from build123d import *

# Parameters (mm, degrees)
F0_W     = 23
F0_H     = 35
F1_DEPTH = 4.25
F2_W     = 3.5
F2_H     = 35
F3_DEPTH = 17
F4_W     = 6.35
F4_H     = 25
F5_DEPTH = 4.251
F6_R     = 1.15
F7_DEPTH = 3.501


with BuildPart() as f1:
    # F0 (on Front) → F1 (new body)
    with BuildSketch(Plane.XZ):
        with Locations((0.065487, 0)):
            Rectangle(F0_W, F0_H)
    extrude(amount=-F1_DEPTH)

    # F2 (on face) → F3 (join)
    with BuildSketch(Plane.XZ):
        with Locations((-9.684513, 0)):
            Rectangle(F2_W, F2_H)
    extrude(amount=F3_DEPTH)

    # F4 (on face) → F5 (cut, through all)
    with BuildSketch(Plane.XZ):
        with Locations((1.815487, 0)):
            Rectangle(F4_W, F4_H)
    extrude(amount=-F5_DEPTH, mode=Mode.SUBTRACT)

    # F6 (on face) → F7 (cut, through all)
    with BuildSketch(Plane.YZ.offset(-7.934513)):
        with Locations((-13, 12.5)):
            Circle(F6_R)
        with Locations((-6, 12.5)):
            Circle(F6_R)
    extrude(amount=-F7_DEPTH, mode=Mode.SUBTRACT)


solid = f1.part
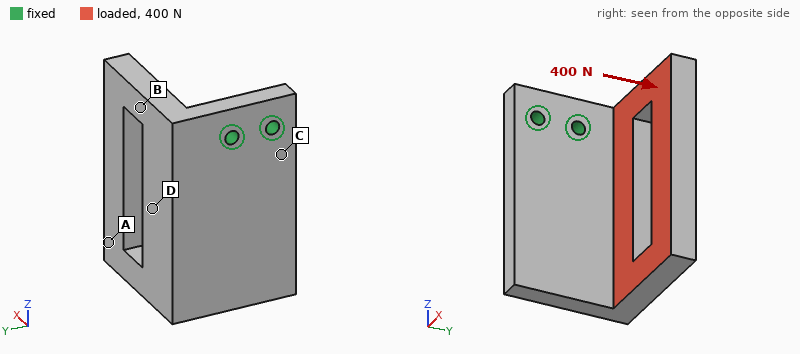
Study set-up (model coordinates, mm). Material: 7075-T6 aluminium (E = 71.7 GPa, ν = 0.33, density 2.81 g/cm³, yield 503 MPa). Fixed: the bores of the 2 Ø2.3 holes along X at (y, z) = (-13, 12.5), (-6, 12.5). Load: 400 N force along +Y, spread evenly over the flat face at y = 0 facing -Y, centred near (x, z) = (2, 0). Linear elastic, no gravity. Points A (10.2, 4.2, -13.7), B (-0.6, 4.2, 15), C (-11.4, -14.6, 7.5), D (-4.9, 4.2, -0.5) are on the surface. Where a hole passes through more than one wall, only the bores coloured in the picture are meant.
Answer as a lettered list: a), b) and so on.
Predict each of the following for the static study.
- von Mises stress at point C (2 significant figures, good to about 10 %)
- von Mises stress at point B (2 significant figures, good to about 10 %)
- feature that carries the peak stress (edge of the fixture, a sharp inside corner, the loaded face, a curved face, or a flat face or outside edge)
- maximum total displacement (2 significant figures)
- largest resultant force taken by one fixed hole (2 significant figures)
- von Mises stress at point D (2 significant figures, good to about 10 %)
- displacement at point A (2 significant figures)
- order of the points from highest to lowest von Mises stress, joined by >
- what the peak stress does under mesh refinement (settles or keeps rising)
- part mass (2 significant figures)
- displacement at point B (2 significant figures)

a) 45 MPa
b) 63 MPa
c) edge of the fixture
d) 0.27 mm
e) 680 N
f) 21 MPa
g) 0.25 mm
h) B > C > D > A
i) keeps rising
j) 13 g
k) 0.085 mm
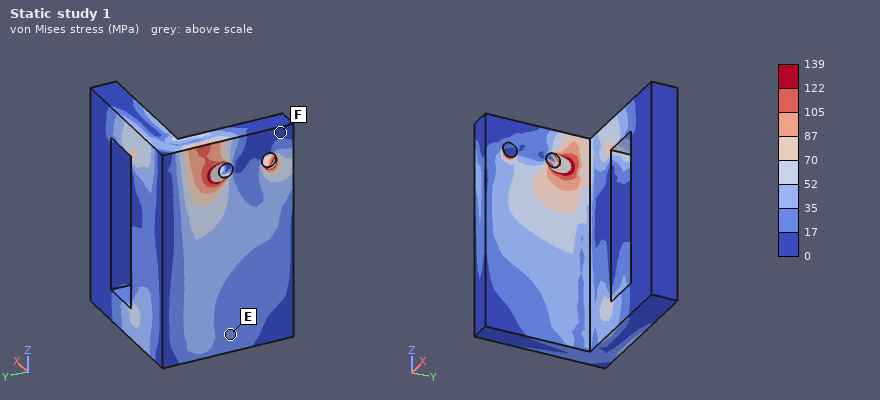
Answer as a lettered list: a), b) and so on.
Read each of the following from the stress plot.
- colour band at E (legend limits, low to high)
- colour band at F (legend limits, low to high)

a) 17 to 35 MPa
b) 0 to 17 MPa
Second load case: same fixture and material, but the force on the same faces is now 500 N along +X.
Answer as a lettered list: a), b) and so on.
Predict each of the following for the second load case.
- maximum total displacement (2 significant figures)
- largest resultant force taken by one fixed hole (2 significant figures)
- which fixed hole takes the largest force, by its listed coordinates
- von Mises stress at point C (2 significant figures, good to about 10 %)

a) 0.29 mm
b) 630 N
c) (-6, 12.5)
d) 80 MPa
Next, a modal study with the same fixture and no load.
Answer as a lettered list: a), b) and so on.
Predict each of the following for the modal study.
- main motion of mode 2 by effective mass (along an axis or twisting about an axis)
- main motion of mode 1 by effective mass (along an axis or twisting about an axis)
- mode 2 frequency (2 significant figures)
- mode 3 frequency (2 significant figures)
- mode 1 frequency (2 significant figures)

a) along Y
b) along X
c) 3100 Hz
d) 6800 Hz
e) 2200 Hz
